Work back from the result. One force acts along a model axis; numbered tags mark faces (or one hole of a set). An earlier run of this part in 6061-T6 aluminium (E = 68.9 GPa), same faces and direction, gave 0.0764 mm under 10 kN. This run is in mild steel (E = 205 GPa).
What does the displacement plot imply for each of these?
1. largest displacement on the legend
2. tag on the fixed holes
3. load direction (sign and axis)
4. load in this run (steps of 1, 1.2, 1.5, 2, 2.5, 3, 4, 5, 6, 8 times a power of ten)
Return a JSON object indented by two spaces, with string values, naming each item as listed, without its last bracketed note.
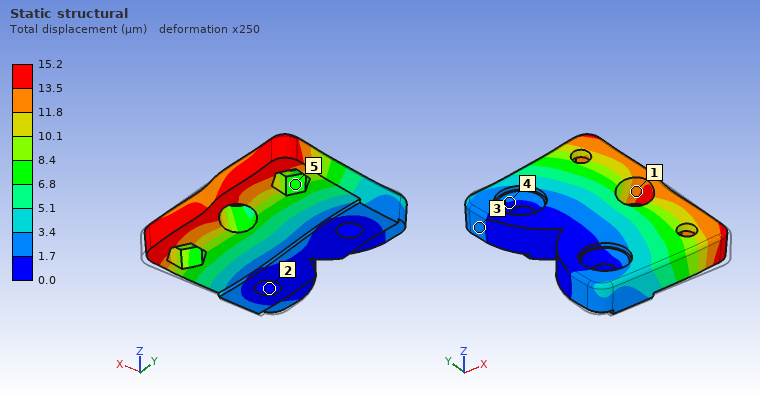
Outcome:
{
  "largest displacement on the legend": "15.2 µm",
  "tag on the fixed holes": "2",
  "load direction": "+Y",
  "load in this run": "6 kN"
}
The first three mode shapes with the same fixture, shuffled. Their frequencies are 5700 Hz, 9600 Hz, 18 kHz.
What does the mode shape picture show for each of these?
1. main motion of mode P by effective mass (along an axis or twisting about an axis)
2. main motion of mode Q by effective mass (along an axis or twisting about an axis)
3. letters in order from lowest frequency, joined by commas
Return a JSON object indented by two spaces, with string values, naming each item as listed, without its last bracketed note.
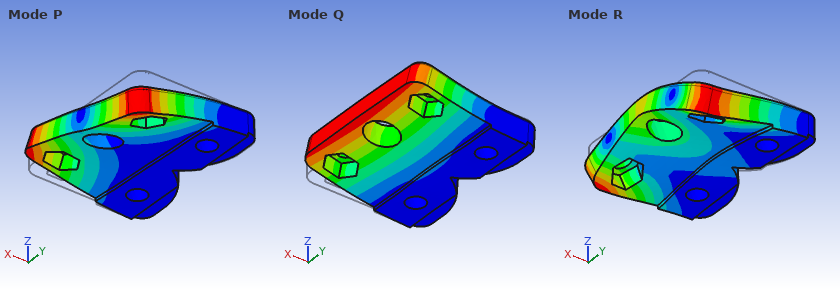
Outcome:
{
  "main motion of mode P by effective mass": "twisting about X",
  "main motion of mode Q by effective mass": "along Z",
  "letters in order from lowest frequency, joined by commas": "Q, P, R"
}
